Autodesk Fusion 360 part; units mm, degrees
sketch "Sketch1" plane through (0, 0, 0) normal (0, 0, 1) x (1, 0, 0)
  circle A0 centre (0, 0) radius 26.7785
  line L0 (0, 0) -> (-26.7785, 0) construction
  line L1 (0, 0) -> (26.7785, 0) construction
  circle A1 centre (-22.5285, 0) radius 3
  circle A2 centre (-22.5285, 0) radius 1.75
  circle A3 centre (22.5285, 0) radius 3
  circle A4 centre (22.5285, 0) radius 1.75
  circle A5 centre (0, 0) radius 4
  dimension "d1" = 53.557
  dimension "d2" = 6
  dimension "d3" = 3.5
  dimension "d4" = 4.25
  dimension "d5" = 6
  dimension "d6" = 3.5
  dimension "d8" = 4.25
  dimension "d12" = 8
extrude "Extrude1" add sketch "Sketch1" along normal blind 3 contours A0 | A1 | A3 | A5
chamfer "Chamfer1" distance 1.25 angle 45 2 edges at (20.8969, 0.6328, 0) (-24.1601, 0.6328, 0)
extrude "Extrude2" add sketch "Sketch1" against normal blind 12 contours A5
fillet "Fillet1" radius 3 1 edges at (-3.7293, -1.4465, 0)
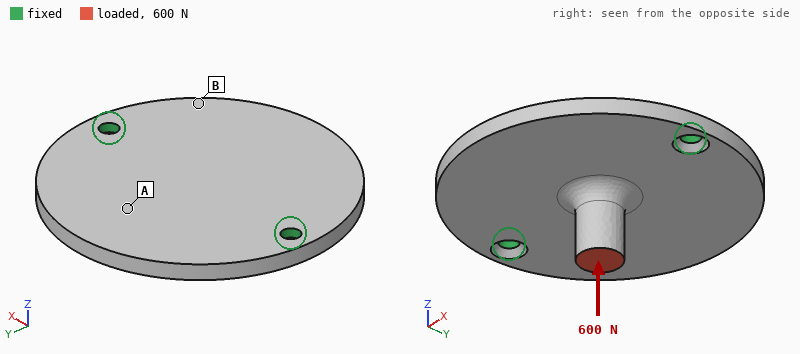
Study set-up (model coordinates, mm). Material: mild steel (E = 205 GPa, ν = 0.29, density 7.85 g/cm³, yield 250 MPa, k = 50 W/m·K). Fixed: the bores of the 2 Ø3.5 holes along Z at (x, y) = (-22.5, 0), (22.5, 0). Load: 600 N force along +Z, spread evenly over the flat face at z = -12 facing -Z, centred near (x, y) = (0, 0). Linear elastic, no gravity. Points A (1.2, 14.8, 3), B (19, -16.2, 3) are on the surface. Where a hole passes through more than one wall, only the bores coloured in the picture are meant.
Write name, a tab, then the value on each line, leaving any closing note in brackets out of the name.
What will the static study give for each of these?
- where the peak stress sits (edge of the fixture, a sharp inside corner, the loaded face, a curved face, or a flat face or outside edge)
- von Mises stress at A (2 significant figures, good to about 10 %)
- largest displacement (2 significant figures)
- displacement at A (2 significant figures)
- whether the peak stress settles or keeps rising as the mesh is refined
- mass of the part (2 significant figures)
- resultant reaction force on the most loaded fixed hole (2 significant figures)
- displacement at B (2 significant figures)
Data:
where the peak stress sits	edge of the fixture
von Mises stress at A	28 MPa
largest displacement	24 µm
displacement at A	22 µm
whether the peak stress settles or keeps rising as the mesh is refined	keeps rising
mass of the part	58 g
resultant reaction force on the most loaded fixed hole	420 N
displacement at B	9.3 µm
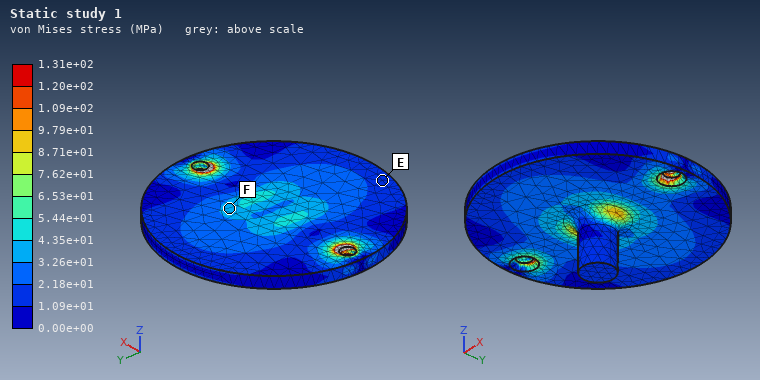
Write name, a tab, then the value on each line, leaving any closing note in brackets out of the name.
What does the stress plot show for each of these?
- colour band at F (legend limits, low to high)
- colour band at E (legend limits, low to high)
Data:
colour band at F	3.26e+01 to 4.35e+01 MPa
colour band at E	1.09e+01 to 2.18e+01 MPa
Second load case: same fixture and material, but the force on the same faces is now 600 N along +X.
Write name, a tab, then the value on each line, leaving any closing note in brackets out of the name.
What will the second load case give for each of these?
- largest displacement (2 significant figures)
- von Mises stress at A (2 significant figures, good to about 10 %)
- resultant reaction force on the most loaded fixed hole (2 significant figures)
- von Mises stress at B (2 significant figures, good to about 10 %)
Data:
largest displacement	28 µm
von Mises stress at A	15 MPa
resultant reaction force on the most loaded fixed hole	380 N
von Mises stress at B	12 MPa
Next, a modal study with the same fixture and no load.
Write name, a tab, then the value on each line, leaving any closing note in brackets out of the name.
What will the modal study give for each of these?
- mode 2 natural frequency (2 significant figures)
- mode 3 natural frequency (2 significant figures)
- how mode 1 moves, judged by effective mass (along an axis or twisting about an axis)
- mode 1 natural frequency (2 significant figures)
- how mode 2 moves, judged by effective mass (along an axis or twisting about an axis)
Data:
mode 2 natural frequency	3600 Hz
mode 3 natural frequency	8100 Hz
how mode 1 moves, judged by effective mass	twisting about X
mode 1 natural frequency	2400 Hz
how mode 2 moves, judged by effective mass	along Z
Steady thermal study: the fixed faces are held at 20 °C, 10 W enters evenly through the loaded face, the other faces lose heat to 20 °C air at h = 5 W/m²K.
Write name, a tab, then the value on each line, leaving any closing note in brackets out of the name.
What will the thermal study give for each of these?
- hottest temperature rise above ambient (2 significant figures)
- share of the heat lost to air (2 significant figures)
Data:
hottest temperature rise above ambient	79 K
share of the heat lost to air	5.0 %
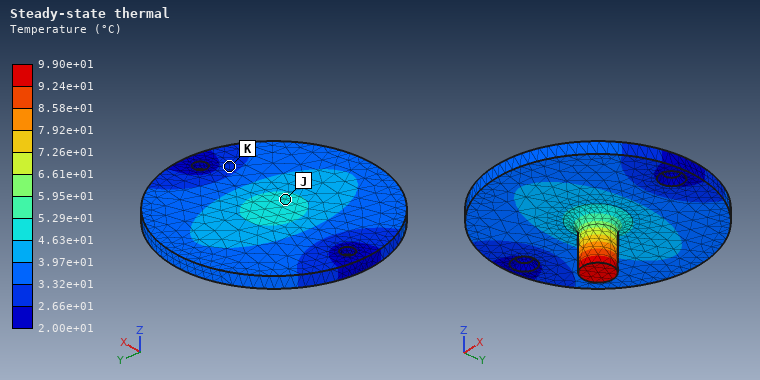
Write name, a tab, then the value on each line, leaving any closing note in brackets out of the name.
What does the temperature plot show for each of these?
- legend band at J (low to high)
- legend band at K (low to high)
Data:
legend band at J	4.63e+01 to 5.29e+01 °C
legend band at K	2.66e+01 to 3.32e+01 °C
